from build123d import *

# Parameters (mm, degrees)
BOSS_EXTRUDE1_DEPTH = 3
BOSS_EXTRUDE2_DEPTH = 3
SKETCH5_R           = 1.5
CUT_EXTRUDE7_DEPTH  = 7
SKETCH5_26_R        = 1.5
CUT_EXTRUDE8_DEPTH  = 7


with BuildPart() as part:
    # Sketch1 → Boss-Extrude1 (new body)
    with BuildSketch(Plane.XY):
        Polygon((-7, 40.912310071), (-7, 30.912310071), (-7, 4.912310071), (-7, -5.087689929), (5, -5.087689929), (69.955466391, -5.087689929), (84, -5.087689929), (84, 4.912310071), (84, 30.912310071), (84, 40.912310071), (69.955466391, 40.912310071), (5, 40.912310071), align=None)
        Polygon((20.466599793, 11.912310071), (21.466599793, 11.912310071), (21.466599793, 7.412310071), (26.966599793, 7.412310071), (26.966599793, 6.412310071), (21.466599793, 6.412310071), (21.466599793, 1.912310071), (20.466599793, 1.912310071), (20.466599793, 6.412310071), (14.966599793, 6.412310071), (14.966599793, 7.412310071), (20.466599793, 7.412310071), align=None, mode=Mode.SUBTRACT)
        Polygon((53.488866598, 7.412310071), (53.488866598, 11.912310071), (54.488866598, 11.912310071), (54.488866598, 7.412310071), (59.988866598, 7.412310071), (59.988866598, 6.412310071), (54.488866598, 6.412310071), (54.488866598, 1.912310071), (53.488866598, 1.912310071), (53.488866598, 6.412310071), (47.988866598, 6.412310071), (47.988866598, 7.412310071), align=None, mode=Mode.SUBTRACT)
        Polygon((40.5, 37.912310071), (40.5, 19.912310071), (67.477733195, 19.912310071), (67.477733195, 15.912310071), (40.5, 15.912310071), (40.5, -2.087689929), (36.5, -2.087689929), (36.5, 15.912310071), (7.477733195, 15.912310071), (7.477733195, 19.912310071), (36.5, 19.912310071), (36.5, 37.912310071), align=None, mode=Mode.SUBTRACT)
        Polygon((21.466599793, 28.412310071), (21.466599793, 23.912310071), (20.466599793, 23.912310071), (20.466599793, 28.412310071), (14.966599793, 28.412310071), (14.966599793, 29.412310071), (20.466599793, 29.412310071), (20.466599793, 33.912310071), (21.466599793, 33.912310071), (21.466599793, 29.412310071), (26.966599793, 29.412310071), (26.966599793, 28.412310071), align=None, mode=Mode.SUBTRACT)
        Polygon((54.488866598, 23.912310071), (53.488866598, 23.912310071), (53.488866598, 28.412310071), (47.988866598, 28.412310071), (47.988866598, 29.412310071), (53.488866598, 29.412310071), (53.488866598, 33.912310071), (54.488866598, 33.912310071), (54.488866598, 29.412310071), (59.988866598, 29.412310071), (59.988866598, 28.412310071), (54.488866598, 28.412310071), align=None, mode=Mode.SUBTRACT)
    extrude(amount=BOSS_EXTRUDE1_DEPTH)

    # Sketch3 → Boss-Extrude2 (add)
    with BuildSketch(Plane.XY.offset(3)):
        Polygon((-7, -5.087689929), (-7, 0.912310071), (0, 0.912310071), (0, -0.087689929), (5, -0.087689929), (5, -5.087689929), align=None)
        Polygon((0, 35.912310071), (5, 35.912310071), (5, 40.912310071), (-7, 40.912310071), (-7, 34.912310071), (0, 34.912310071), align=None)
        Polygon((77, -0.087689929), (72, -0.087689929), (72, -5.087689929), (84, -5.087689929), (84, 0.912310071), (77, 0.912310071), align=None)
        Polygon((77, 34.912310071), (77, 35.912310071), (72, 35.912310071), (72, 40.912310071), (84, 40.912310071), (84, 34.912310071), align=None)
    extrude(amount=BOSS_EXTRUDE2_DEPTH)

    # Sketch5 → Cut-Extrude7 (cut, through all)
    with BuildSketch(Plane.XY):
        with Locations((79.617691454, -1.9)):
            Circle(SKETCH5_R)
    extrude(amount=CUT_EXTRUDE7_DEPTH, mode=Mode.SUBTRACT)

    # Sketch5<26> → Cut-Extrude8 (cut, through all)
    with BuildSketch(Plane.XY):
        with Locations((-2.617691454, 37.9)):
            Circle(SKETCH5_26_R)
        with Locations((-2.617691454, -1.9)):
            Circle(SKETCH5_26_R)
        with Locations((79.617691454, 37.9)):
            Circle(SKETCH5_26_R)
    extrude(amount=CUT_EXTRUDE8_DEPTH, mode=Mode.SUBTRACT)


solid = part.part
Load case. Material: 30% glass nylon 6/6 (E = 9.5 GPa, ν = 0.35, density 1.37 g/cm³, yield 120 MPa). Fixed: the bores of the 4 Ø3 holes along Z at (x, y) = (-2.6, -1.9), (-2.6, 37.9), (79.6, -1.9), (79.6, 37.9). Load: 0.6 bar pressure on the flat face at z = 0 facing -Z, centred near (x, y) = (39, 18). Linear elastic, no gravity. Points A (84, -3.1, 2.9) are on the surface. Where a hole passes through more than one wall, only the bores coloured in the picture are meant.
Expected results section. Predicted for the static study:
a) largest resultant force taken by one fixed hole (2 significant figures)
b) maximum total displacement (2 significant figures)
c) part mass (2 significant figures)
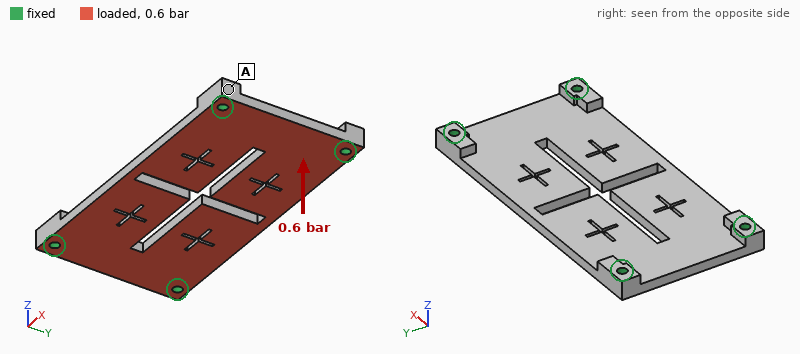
59 N
0.55 mm
16 g
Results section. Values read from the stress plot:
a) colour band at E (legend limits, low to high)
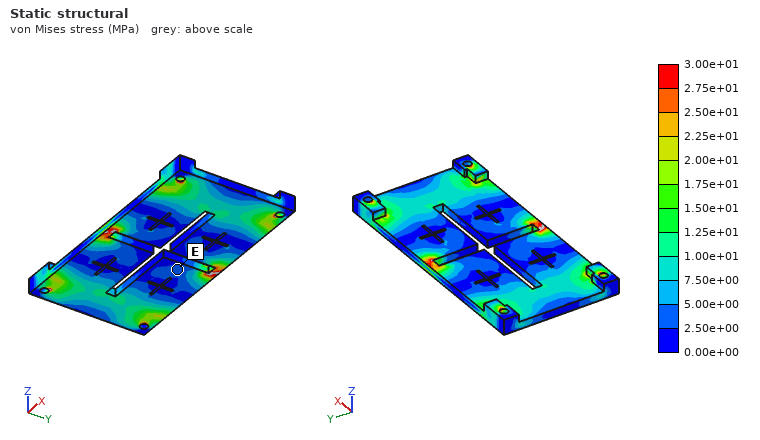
2.50e+00 to 5.00e+00 MPa
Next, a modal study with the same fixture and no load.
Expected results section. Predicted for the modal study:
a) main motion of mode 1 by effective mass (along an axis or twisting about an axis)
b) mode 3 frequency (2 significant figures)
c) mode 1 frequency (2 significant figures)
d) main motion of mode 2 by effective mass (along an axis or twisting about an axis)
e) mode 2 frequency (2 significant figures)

along Z
2000 Hz
1100 Hz
twisting about X
1300 Hz
